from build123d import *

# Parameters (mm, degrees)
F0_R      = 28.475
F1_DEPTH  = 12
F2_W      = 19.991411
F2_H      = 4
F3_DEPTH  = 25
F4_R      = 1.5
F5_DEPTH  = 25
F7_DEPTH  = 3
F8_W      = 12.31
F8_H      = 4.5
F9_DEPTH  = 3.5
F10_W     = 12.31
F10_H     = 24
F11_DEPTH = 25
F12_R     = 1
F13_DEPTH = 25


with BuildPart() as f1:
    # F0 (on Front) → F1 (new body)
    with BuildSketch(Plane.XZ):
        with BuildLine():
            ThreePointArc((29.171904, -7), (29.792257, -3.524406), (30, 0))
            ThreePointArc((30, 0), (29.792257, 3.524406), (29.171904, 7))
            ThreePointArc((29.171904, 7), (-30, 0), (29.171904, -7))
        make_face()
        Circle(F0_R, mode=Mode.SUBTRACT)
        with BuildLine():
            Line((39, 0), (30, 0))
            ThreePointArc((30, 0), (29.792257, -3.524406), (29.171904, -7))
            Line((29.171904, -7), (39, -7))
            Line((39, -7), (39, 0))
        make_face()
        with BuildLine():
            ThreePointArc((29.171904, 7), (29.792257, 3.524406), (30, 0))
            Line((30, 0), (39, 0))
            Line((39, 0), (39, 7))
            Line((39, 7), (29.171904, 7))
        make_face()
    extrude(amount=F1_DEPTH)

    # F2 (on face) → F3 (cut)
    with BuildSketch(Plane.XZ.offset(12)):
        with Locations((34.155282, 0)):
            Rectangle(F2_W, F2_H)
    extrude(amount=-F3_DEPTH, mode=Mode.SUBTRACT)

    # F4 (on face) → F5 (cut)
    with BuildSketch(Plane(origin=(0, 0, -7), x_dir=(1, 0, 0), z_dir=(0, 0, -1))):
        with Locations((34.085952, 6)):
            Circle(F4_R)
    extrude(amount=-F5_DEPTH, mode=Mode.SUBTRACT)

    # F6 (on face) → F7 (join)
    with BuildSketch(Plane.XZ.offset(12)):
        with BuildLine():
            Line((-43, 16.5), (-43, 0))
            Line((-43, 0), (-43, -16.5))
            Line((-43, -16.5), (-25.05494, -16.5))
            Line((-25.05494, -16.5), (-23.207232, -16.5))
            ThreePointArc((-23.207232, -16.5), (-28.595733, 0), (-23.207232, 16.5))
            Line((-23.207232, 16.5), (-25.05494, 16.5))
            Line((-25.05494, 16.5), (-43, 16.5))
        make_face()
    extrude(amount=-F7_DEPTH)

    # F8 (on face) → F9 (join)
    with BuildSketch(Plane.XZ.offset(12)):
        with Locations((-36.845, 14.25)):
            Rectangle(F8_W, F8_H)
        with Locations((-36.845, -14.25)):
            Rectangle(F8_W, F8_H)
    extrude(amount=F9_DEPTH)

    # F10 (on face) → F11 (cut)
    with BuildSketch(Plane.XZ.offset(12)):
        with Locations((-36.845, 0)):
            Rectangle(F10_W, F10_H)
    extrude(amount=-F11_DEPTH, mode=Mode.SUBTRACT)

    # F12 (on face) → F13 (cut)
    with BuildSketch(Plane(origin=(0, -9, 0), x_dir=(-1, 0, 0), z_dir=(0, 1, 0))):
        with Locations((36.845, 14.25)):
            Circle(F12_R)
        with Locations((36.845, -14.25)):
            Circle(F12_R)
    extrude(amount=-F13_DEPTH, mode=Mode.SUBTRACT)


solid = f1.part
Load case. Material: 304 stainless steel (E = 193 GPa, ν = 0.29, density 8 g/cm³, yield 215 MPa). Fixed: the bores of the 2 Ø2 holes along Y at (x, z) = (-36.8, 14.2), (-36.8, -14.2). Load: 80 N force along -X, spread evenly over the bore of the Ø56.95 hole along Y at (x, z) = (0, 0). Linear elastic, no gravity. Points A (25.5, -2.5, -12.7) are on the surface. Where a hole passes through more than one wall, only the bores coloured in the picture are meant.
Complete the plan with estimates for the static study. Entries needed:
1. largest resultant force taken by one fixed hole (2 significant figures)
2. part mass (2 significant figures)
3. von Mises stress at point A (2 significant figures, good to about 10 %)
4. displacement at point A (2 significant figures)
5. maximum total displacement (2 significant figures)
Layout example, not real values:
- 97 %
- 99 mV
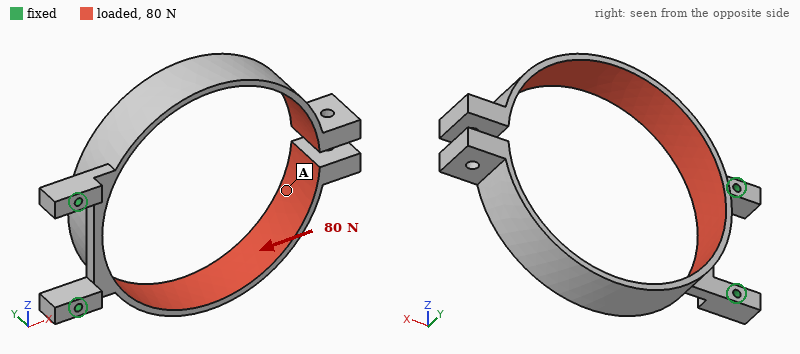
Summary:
- 45 N
- 42 g
- 6.4 MPa
- 0.22 mm
- 0.37 mm
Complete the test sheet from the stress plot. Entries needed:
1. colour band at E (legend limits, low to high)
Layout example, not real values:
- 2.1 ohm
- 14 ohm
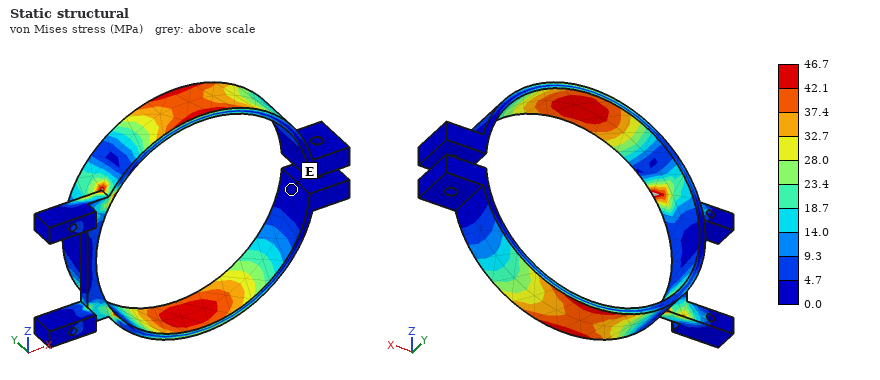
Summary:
- 0.0 to 4.7 MPa
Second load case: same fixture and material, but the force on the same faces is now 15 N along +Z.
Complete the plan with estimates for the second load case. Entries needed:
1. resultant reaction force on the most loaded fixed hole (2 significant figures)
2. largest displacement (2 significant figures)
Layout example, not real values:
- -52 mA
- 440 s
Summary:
- 12 N
- 0.39 mm
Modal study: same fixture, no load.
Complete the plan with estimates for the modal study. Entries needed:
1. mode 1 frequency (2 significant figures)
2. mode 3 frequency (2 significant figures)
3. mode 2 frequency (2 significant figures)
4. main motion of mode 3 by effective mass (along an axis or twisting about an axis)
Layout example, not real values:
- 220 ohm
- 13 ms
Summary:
- 150 Hz
- 220 Hz
- 150 Hz
- along Y
